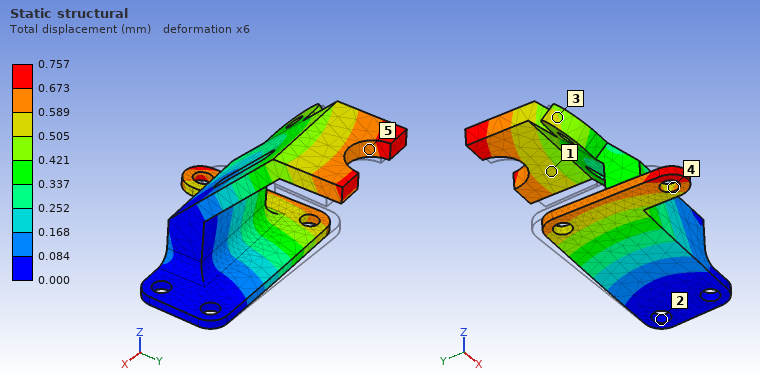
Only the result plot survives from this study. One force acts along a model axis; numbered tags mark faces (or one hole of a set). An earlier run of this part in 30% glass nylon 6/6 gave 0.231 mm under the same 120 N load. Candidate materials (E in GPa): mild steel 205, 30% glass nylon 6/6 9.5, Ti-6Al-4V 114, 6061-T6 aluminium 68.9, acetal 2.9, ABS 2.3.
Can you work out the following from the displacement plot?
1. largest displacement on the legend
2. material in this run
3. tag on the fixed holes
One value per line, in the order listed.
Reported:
0.757 mm
acetal
2
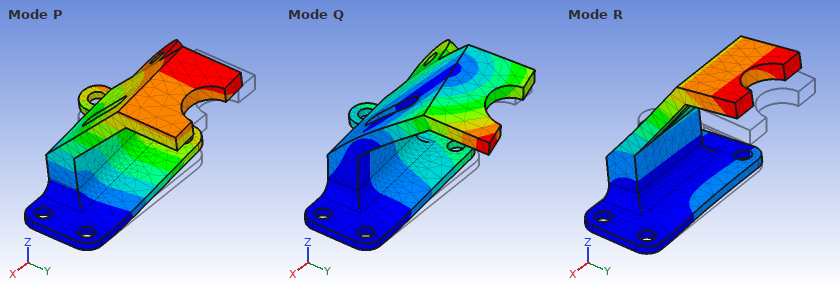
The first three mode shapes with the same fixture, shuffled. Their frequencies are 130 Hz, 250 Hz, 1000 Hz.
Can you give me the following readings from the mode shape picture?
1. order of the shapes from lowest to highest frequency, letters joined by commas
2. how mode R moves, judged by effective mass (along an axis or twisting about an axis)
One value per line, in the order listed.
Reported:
P, R, Q
along Y
